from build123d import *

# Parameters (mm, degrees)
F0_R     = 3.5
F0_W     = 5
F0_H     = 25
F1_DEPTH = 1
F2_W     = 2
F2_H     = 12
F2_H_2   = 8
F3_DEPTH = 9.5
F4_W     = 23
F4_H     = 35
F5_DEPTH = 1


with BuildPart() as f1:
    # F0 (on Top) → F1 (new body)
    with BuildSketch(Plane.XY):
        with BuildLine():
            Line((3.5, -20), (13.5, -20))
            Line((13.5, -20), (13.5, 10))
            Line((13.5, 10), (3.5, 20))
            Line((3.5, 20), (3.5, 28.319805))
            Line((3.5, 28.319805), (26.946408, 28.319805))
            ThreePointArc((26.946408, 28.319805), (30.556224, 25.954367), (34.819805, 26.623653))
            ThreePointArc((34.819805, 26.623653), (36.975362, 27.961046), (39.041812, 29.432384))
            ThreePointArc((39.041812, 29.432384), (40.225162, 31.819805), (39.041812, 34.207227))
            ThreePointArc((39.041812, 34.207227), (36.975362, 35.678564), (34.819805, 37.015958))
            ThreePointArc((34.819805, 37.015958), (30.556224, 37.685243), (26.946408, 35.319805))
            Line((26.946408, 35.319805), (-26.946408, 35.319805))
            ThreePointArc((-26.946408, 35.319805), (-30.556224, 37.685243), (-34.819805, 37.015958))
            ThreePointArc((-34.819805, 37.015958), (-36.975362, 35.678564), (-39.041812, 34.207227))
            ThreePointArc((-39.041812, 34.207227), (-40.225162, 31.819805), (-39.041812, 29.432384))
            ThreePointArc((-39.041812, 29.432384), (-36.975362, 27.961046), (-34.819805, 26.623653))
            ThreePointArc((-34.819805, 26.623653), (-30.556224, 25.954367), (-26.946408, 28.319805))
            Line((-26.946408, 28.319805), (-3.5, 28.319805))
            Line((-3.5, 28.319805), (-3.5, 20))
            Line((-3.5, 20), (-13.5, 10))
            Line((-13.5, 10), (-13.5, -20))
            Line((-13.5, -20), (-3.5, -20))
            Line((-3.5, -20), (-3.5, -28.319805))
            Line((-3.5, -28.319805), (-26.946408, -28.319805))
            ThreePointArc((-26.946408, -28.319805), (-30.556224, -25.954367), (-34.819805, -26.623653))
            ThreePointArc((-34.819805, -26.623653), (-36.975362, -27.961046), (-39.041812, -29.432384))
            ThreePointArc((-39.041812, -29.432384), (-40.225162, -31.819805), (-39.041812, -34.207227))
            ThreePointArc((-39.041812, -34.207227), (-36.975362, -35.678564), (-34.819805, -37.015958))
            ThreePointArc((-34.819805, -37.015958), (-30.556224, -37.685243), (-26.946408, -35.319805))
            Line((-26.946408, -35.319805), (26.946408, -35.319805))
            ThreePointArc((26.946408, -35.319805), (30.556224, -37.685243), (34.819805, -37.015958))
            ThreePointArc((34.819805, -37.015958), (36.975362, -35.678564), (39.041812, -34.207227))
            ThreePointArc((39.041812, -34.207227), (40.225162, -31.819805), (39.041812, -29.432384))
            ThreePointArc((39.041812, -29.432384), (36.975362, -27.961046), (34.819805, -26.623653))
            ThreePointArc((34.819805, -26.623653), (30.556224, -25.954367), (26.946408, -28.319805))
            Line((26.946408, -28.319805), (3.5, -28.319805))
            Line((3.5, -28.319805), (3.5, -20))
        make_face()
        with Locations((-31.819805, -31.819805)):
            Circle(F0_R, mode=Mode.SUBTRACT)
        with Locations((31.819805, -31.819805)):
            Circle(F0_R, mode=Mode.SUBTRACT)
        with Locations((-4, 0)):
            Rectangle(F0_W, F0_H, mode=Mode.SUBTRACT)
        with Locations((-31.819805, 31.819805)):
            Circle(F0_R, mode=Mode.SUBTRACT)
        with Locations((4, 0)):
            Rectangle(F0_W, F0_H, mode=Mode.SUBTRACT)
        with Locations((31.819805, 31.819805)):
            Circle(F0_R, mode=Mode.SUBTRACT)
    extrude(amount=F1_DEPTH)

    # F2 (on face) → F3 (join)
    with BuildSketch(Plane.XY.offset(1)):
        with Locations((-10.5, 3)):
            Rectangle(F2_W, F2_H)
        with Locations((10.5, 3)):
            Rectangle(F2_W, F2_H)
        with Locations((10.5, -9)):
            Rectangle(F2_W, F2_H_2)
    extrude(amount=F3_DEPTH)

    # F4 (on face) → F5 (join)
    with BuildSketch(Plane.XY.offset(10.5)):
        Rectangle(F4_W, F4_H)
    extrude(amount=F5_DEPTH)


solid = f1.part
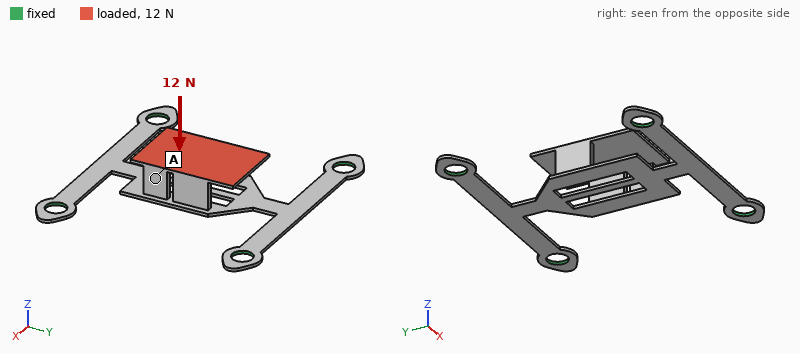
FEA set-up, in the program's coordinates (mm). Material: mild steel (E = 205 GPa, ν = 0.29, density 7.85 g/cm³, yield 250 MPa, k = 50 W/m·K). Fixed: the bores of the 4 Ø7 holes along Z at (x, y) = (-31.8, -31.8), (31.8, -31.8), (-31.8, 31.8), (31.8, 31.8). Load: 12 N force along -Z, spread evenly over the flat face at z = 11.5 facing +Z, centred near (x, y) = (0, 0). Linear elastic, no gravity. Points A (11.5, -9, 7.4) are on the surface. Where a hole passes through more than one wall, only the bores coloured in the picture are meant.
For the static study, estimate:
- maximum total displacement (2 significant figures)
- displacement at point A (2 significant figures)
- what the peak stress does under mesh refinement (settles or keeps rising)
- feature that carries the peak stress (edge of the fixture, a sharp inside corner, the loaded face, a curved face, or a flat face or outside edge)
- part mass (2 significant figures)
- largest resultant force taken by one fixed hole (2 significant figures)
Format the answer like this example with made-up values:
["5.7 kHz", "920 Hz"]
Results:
["0.13 mm", "0.11 mm", "keeps rising", "a sharp inside corner", "26 g", "3.2 N"]
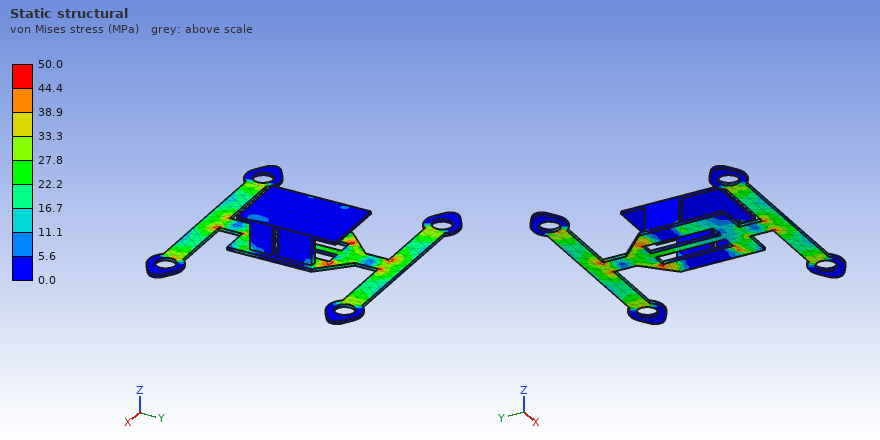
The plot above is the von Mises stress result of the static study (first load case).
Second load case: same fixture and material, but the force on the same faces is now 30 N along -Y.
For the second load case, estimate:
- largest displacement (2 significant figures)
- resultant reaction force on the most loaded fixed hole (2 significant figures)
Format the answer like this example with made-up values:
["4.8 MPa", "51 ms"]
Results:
["0.11 mm", "8.4 N"]
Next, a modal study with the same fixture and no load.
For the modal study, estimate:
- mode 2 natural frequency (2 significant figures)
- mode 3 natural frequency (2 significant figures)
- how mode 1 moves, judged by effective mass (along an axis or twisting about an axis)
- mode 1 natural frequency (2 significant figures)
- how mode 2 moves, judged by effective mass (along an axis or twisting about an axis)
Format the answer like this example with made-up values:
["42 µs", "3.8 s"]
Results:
["480 Hz", "830 Hz", "along Z", "390 Hz", "along X"]
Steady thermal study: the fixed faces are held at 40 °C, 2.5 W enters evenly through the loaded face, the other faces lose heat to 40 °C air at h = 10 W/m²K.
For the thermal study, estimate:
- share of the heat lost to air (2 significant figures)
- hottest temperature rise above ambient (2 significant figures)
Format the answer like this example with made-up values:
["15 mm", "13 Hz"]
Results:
["68 %", "59 K"]
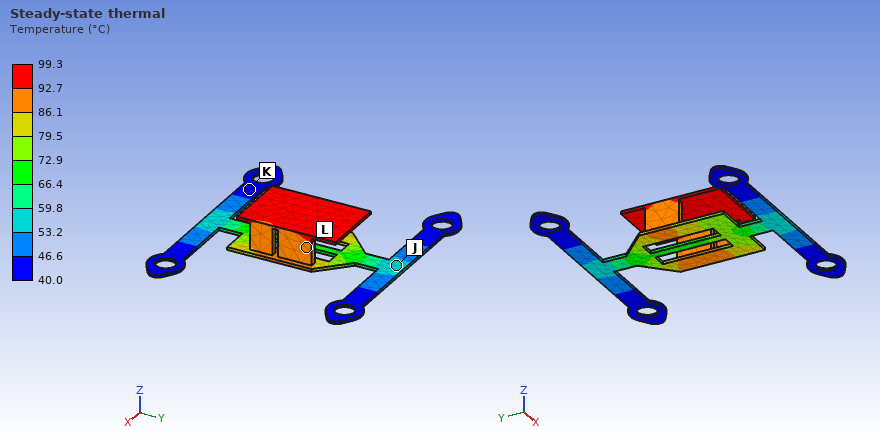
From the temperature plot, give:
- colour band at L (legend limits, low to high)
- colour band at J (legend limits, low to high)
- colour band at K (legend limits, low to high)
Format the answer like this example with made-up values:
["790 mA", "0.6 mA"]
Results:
["86.1 to 92.7 °C", "53.2 to 59.8 °C", "40.0 to 46.6 °C"]
